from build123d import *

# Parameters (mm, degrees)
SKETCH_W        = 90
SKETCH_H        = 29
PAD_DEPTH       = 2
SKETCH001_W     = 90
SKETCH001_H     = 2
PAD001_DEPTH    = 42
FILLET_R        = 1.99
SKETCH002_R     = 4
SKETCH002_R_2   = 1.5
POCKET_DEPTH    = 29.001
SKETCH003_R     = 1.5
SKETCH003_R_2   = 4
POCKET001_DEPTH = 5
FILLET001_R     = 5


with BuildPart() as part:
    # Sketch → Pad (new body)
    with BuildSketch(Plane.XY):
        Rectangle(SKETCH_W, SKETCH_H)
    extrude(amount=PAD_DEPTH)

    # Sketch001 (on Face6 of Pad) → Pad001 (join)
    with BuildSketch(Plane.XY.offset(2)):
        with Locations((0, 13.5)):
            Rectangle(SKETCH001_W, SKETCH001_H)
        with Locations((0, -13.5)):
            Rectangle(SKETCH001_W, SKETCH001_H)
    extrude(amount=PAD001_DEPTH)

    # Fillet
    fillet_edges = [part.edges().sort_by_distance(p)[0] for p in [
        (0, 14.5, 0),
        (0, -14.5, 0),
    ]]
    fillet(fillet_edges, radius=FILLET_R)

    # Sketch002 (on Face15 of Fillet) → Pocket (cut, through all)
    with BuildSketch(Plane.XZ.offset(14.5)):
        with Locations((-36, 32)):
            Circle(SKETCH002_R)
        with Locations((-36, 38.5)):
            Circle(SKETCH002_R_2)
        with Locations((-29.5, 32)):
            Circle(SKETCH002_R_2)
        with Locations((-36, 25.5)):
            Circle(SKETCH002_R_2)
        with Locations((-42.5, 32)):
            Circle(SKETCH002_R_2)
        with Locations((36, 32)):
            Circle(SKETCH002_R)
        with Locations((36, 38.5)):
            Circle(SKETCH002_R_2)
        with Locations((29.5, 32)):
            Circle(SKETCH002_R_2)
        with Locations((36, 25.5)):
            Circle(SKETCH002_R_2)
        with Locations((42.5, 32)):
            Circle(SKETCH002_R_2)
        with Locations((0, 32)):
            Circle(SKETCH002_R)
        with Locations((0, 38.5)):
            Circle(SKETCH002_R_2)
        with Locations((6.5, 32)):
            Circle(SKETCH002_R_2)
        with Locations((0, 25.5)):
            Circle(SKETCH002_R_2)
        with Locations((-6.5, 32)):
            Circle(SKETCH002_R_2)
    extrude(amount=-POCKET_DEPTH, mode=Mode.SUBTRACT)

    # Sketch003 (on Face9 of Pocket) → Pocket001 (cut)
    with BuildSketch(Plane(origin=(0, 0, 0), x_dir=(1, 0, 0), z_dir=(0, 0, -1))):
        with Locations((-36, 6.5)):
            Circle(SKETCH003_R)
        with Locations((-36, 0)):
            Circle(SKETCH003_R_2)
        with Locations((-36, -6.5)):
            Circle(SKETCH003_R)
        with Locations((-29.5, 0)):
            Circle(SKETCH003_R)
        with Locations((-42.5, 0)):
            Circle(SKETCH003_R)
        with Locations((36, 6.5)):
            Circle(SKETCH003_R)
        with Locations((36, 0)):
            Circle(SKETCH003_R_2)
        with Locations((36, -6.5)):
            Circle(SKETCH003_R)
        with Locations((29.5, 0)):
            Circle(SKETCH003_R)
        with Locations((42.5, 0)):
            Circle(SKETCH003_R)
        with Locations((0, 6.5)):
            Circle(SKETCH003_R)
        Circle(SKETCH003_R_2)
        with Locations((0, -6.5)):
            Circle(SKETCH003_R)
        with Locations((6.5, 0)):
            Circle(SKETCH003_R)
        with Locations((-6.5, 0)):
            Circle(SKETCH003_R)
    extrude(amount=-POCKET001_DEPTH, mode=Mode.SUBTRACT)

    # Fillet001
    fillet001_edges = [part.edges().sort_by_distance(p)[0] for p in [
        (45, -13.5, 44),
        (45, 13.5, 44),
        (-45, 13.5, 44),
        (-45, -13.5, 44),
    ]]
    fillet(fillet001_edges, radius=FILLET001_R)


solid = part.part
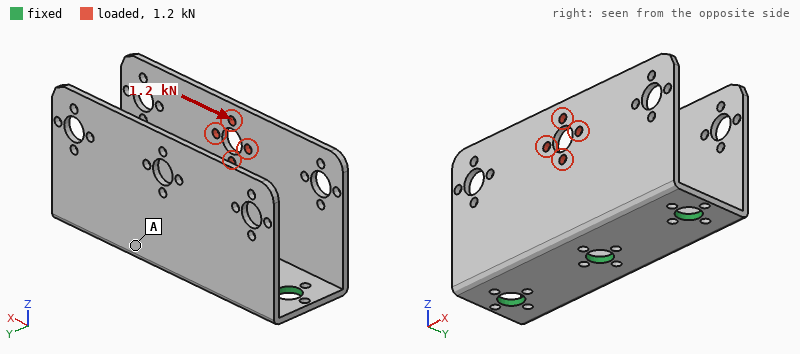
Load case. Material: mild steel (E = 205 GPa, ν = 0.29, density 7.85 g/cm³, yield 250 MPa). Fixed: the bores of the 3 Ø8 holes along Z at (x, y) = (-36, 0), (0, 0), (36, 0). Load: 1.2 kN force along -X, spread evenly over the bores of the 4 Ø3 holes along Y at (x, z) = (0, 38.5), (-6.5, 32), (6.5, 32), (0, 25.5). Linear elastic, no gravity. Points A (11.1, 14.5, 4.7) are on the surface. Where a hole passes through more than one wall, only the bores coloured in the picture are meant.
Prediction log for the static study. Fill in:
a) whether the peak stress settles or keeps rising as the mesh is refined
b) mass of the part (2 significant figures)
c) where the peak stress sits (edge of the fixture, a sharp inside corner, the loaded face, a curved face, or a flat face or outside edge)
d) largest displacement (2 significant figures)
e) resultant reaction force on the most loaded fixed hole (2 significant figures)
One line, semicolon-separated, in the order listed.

keeps rising; 150 g; a sharp inside corner; 0.21 mm; 640 N
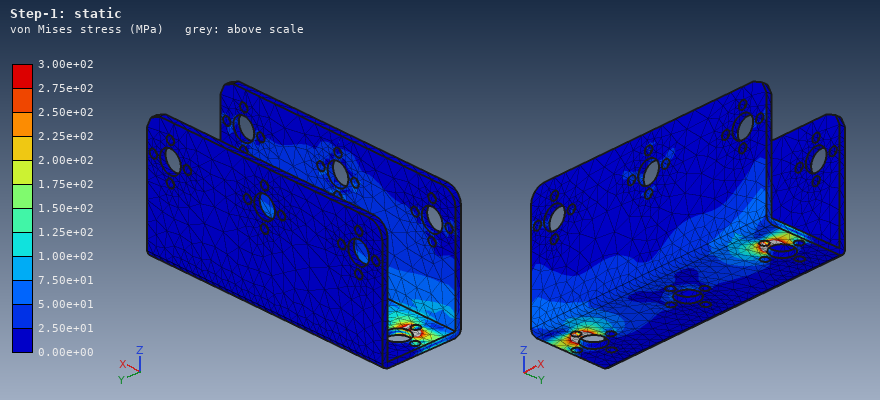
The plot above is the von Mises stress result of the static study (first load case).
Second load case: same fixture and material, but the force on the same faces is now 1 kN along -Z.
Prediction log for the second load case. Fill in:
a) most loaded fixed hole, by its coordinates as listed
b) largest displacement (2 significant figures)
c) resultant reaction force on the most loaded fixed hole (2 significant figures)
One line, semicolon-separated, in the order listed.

(0, 0); 0.27 mm; 410 N
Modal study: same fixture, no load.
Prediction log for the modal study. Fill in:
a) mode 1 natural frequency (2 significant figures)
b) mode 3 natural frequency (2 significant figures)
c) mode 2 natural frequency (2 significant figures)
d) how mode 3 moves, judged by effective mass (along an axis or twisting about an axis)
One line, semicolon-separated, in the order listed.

650 Hz; 1100 Hz; 660 Hz; twisting about Z
